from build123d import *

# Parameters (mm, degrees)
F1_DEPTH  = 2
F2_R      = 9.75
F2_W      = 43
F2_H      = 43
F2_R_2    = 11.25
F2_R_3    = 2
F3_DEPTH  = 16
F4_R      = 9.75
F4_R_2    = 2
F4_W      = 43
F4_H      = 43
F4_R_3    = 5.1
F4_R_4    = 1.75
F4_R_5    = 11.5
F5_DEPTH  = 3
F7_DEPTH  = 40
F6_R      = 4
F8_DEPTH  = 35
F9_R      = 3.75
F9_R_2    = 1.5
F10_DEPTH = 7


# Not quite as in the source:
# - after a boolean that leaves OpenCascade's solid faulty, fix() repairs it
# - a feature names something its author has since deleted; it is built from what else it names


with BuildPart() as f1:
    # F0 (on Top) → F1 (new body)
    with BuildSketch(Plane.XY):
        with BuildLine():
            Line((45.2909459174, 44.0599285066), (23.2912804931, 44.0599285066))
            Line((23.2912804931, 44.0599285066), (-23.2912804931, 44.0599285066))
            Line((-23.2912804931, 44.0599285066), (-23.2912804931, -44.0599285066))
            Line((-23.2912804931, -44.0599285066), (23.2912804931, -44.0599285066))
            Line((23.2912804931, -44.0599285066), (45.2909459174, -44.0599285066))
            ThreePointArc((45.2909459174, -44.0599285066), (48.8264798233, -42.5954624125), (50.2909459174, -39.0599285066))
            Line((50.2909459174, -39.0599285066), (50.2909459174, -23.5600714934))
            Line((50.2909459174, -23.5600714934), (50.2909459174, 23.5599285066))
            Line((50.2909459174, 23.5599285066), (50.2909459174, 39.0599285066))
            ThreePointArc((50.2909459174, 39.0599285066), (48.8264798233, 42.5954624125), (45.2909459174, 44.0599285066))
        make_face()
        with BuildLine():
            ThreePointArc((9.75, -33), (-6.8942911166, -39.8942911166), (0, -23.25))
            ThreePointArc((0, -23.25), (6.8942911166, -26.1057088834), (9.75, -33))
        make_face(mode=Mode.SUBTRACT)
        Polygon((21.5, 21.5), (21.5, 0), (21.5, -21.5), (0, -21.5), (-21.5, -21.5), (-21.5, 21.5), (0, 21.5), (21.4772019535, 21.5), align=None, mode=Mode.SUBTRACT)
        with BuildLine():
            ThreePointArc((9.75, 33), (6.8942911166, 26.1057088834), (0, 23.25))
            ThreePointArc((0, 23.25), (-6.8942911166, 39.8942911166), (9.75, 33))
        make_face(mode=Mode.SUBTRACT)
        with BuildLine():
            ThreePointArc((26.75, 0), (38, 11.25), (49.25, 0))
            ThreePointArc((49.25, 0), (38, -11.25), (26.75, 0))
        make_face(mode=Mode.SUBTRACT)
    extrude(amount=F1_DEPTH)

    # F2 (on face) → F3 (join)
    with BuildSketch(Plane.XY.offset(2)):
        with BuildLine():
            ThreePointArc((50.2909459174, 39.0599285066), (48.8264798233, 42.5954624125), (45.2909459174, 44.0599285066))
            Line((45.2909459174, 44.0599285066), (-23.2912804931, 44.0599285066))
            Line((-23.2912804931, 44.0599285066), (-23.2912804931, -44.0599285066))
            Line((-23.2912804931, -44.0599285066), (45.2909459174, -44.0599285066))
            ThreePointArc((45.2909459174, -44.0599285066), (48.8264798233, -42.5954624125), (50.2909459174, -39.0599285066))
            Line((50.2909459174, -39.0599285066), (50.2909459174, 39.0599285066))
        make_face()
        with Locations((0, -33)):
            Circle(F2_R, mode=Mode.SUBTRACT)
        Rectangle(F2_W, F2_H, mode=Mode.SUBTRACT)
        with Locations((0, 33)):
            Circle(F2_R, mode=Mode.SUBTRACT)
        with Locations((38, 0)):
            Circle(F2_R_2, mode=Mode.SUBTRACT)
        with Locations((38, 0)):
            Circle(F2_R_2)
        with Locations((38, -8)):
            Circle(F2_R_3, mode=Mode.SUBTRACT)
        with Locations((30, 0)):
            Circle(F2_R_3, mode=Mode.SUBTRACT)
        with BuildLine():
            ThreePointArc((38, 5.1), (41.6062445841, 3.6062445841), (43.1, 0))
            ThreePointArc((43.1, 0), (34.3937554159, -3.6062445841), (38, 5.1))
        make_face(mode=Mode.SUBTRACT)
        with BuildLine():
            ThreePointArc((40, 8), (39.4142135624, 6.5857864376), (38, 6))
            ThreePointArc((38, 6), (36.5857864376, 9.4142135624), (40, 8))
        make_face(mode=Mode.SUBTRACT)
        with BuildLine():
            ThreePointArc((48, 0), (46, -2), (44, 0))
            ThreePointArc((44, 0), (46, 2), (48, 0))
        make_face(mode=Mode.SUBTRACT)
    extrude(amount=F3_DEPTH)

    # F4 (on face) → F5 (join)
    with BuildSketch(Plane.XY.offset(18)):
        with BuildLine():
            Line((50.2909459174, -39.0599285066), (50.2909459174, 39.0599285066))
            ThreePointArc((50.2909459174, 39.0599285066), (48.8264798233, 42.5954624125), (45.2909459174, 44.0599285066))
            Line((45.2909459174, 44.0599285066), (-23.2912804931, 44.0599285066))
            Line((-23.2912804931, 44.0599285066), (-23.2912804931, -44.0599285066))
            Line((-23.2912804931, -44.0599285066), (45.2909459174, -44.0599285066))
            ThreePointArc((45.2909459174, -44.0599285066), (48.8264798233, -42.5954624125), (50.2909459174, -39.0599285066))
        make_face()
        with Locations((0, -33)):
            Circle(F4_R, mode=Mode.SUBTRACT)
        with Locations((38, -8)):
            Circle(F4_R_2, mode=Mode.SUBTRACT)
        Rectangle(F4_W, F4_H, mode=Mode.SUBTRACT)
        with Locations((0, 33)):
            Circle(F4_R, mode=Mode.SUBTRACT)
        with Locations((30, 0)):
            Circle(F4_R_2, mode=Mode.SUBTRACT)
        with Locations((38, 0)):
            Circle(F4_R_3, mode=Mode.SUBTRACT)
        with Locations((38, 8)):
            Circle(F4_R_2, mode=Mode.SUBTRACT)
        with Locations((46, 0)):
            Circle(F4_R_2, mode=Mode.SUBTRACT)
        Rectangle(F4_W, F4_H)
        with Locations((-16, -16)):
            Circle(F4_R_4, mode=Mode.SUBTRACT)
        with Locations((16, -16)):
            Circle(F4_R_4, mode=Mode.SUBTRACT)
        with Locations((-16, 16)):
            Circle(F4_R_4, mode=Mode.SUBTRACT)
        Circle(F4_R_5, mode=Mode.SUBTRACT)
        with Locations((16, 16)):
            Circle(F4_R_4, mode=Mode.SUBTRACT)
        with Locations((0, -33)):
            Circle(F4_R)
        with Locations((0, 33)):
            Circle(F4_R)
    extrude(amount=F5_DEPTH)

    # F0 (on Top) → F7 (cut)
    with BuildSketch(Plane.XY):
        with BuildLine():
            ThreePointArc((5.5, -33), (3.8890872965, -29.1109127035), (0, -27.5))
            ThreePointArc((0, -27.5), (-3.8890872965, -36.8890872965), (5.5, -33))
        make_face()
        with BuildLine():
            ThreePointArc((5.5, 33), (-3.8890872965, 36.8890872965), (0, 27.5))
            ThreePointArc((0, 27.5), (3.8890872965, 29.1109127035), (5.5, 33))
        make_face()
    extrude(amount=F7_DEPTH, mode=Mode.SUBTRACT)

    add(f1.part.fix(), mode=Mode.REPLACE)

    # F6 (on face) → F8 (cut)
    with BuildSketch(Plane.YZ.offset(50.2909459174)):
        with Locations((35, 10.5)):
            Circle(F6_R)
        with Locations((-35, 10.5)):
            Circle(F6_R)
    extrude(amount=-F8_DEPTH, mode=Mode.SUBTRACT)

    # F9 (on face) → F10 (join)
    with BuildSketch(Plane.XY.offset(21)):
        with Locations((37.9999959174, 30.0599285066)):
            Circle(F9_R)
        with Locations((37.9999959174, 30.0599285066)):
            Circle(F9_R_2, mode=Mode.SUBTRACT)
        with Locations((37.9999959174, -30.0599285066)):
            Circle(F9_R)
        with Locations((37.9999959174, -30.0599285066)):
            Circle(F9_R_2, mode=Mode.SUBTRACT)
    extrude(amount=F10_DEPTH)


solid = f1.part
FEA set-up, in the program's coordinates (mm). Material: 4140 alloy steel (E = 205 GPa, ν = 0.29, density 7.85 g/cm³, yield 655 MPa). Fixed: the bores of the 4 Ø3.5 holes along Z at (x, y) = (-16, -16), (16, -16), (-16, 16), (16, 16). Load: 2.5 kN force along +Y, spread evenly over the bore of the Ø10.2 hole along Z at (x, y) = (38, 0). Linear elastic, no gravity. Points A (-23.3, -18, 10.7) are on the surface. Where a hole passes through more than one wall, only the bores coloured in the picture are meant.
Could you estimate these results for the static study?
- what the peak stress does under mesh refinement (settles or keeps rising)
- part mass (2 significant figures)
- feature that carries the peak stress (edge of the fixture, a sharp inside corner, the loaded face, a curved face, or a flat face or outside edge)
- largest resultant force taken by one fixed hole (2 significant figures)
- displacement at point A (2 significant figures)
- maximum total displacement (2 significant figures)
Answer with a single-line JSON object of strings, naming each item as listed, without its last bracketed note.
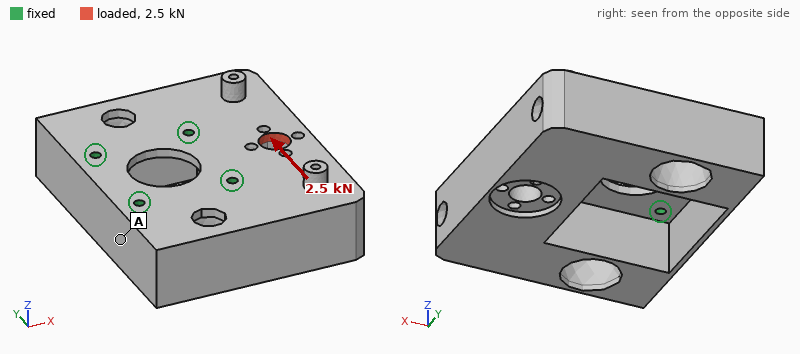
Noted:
{"what the peak stress does under mesh refinement": "keeps rising", "part mass": "660 g", "feature that carries the peak stress": "edge of the fixture", "largest resultant force taken by one fixed hole": "1.7 kN", "displacement at point A": "0.98 µm", "maximum total displacement": "5.8 µm"}
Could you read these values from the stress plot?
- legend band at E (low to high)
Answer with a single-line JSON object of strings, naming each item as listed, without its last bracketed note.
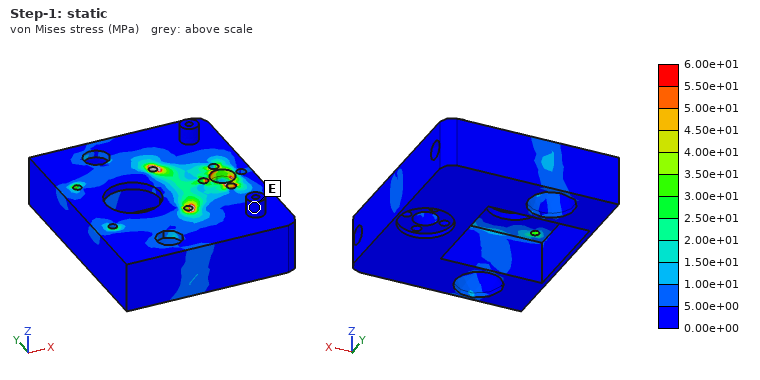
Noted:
{"legend band at E": "0.00e+00 to 5.00e+00 MPa"}
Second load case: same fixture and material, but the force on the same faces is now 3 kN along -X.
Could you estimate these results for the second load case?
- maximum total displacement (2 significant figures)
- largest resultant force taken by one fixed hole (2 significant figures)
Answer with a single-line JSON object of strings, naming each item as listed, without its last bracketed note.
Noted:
{"maximum total displacement": "5.7 µm", "largest resultant force taken by one fixed hole": "1.3 kN"}
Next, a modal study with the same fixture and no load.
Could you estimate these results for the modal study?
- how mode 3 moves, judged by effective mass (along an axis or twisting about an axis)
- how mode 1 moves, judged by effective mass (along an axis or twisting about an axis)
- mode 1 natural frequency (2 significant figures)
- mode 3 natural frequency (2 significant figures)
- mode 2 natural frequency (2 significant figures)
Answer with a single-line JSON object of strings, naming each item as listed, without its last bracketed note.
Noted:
{"how mode 3 moves, judged by effective mass": "along Y", "how mode 1 moves, judged by effective mass": "along Z", "mode 1 natural frequency": "2700 Hz", "mode 3 natural frequency": "5400 Hz", "mode 2 natural frequency": "2900 Hz"}
